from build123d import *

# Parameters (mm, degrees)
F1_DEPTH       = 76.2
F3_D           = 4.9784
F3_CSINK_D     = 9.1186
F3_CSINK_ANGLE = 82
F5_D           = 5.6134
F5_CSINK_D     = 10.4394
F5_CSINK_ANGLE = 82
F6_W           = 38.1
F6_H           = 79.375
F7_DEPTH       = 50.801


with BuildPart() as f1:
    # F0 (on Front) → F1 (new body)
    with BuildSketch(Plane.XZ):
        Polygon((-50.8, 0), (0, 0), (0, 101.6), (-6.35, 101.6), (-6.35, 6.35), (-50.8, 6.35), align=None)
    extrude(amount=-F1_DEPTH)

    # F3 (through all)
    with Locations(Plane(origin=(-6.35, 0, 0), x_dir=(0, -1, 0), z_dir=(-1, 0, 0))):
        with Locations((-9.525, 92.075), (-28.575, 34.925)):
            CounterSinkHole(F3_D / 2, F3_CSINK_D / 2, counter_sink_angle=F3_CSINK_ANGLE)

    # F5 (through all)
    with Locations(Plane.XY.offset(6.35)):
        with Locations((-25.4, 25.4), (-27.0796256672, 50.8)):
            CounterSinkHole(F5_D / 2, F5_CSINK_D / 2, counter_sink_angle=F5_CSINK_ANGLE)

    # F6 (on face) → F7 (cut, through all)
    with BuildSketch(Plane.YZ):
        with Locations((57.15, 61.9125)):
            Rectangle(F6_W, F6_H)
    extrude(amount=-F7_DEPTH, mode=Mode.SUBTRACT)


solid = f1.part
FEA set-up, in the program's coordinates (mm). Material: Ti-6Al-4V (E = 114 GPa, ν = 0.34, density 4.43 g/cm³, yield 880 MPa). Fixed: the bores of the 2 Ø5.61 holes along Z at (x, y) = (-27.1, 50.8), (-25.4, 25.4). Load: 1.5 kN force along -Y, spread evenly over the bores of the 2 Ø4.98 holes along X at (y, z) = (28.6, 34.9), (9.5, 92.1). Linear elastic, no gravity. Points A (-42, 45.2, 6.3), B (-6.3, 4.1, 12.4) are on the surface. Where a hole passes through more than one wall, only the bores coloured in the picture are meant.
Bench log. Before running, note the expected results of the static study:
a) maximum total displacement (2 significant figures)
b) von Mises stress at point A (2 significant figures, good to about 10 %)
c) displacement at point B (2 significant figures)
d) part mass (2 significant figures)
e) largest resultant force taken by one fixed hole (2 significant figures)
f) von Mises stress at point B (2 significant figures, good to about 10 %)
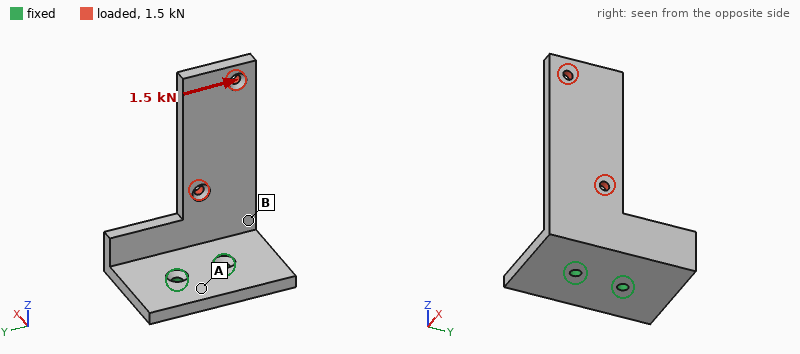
0.59 mm
28 MPa
0.15 mm
220 g
3.4 kN
59 MPa
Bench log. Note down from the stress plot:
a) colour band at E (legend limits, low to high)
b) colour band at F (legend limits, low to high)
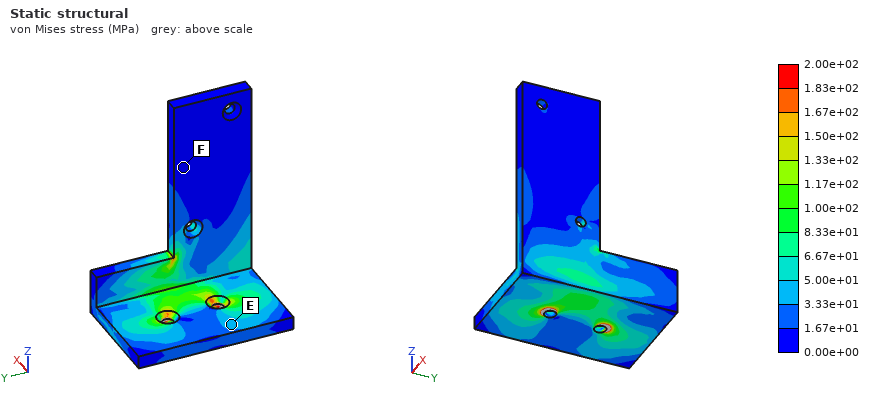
3.33e+01 to 5.00e+01 MPa
0.00e+00 to 1.67e+01 MPa
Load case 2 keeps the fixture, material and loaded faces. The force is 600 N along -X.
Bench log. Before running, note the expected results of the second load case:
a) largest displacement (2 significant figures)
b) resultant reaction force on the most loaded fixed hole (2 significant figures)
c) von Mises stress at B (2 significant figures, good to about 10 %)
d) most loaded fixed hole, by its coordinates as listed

1.6 mm
680 N
86 MPa
(-25.4, 25.4)
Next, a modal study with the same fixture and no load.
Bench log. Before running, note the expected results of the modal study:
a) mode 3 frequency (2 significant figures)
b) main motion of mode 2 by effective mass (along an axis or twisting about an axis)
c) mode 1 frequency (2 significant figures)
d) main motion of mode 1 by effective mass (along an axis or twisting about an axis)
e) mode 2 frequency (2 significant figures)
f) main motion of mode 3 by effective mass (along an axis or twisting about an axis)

2000 Hz
along Y
430 Hz
along X
1100 Hz
along Z
